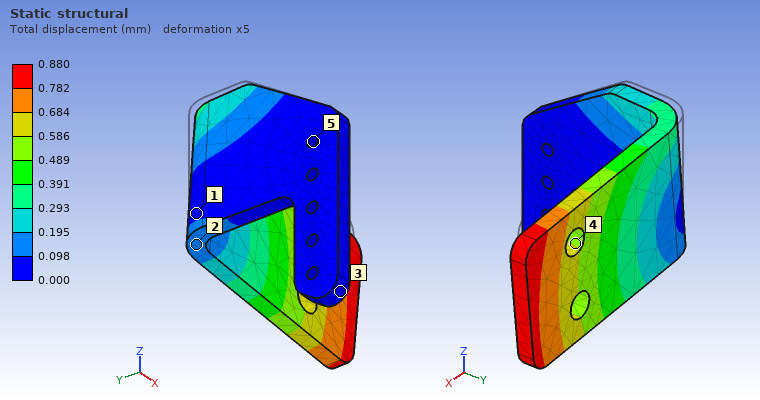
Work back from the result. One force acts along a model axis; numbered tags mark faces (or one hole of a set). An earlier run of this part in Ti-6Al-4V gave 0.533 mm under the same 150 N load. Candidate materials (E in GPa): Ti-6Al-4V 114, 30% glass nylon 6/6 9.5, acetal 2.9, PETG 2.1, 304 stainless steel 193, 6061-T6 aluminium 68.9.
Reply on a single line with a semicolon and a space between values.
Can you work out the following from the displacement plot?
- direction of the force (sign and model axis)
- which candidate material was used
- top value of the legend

-Z; 6061-T6 aluminium; 0.880 mm
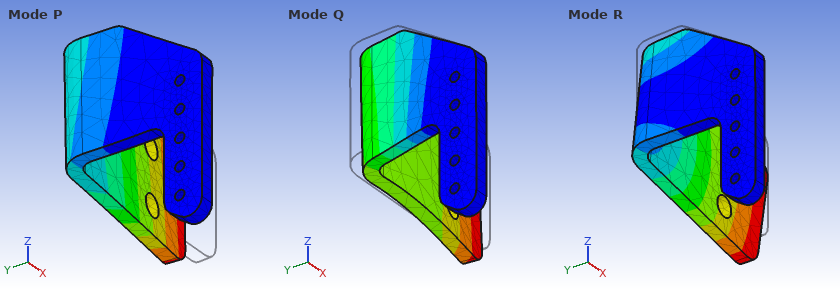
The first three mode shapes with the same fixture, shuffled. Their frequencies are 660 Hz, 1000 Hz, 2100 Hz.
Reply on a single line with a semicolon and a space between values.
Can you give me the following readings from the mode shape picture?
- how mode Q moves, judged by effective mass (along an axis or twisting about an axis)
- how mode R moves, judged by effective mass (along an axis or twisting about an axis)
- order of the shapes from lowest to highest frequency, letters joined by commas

along X; along Z; P, R, Q
